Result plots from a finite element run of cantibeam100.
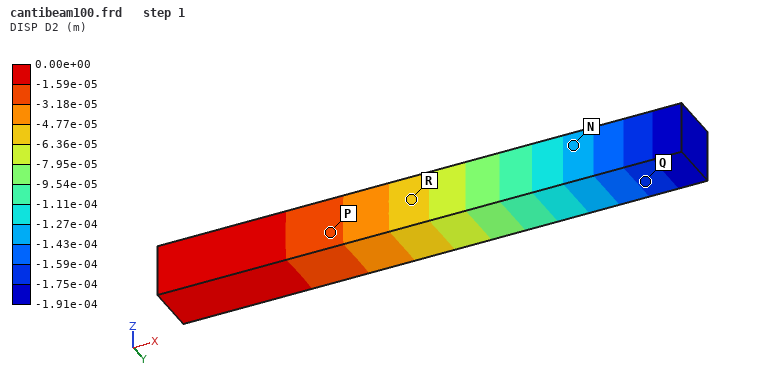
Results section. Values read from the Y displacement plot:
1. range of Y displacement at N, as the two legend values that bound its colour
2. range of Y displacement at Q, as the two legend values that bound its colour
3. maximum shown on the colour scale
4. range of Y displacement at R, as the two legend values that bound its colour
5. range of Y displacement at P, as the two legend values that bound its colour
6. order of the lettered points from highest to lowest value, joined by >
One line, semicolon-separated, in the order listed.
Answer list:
-1.43e-04 to -1.27e-04 m; -1.75e-04 to -1.59e-04 m; 0.00e+00 m; -6.36e-05 to -4.77e-05 m; -3.18e-05 to -1.59e-05 m; P > R > N > Q
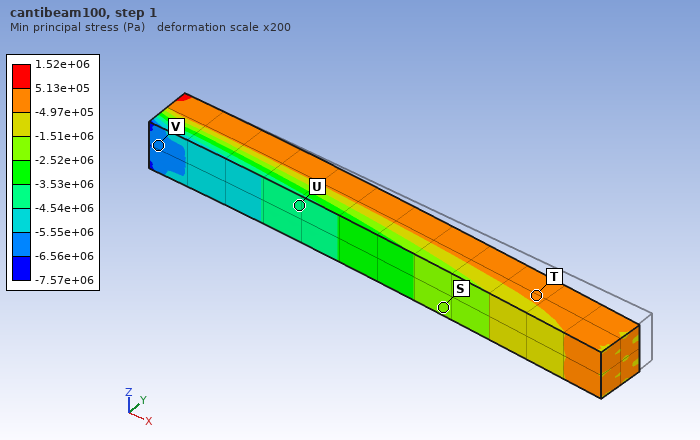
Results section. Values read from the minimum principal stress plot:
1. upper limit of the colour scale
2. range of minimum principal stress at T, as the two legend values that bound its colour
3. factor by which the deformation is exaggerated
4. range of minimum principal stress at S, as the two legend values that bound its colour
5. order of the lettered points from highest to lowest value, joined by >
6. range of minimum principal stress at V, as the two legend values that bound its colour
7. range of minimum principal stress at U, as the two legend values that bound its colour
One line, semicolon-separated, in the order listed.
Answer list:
1.52e+06 Pa; -4.97e+05 to 5.13e+05 Pa; 200; -2.52e+06 to -1.51e+06 Pa; T > S > U > V; -6.56e+06 to -5.55e+06 Pa; -4.54e+06 to -3.53e+06 Pa
